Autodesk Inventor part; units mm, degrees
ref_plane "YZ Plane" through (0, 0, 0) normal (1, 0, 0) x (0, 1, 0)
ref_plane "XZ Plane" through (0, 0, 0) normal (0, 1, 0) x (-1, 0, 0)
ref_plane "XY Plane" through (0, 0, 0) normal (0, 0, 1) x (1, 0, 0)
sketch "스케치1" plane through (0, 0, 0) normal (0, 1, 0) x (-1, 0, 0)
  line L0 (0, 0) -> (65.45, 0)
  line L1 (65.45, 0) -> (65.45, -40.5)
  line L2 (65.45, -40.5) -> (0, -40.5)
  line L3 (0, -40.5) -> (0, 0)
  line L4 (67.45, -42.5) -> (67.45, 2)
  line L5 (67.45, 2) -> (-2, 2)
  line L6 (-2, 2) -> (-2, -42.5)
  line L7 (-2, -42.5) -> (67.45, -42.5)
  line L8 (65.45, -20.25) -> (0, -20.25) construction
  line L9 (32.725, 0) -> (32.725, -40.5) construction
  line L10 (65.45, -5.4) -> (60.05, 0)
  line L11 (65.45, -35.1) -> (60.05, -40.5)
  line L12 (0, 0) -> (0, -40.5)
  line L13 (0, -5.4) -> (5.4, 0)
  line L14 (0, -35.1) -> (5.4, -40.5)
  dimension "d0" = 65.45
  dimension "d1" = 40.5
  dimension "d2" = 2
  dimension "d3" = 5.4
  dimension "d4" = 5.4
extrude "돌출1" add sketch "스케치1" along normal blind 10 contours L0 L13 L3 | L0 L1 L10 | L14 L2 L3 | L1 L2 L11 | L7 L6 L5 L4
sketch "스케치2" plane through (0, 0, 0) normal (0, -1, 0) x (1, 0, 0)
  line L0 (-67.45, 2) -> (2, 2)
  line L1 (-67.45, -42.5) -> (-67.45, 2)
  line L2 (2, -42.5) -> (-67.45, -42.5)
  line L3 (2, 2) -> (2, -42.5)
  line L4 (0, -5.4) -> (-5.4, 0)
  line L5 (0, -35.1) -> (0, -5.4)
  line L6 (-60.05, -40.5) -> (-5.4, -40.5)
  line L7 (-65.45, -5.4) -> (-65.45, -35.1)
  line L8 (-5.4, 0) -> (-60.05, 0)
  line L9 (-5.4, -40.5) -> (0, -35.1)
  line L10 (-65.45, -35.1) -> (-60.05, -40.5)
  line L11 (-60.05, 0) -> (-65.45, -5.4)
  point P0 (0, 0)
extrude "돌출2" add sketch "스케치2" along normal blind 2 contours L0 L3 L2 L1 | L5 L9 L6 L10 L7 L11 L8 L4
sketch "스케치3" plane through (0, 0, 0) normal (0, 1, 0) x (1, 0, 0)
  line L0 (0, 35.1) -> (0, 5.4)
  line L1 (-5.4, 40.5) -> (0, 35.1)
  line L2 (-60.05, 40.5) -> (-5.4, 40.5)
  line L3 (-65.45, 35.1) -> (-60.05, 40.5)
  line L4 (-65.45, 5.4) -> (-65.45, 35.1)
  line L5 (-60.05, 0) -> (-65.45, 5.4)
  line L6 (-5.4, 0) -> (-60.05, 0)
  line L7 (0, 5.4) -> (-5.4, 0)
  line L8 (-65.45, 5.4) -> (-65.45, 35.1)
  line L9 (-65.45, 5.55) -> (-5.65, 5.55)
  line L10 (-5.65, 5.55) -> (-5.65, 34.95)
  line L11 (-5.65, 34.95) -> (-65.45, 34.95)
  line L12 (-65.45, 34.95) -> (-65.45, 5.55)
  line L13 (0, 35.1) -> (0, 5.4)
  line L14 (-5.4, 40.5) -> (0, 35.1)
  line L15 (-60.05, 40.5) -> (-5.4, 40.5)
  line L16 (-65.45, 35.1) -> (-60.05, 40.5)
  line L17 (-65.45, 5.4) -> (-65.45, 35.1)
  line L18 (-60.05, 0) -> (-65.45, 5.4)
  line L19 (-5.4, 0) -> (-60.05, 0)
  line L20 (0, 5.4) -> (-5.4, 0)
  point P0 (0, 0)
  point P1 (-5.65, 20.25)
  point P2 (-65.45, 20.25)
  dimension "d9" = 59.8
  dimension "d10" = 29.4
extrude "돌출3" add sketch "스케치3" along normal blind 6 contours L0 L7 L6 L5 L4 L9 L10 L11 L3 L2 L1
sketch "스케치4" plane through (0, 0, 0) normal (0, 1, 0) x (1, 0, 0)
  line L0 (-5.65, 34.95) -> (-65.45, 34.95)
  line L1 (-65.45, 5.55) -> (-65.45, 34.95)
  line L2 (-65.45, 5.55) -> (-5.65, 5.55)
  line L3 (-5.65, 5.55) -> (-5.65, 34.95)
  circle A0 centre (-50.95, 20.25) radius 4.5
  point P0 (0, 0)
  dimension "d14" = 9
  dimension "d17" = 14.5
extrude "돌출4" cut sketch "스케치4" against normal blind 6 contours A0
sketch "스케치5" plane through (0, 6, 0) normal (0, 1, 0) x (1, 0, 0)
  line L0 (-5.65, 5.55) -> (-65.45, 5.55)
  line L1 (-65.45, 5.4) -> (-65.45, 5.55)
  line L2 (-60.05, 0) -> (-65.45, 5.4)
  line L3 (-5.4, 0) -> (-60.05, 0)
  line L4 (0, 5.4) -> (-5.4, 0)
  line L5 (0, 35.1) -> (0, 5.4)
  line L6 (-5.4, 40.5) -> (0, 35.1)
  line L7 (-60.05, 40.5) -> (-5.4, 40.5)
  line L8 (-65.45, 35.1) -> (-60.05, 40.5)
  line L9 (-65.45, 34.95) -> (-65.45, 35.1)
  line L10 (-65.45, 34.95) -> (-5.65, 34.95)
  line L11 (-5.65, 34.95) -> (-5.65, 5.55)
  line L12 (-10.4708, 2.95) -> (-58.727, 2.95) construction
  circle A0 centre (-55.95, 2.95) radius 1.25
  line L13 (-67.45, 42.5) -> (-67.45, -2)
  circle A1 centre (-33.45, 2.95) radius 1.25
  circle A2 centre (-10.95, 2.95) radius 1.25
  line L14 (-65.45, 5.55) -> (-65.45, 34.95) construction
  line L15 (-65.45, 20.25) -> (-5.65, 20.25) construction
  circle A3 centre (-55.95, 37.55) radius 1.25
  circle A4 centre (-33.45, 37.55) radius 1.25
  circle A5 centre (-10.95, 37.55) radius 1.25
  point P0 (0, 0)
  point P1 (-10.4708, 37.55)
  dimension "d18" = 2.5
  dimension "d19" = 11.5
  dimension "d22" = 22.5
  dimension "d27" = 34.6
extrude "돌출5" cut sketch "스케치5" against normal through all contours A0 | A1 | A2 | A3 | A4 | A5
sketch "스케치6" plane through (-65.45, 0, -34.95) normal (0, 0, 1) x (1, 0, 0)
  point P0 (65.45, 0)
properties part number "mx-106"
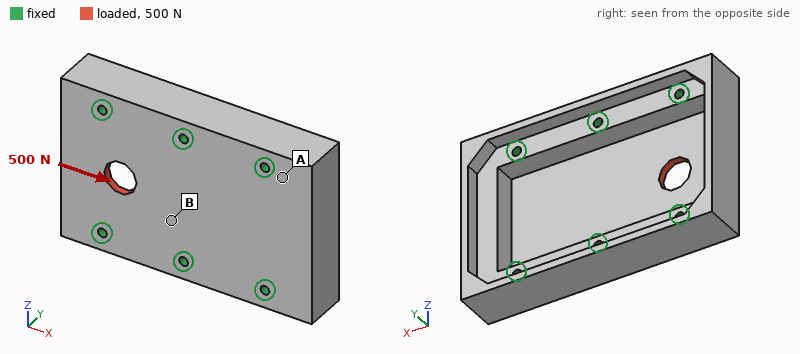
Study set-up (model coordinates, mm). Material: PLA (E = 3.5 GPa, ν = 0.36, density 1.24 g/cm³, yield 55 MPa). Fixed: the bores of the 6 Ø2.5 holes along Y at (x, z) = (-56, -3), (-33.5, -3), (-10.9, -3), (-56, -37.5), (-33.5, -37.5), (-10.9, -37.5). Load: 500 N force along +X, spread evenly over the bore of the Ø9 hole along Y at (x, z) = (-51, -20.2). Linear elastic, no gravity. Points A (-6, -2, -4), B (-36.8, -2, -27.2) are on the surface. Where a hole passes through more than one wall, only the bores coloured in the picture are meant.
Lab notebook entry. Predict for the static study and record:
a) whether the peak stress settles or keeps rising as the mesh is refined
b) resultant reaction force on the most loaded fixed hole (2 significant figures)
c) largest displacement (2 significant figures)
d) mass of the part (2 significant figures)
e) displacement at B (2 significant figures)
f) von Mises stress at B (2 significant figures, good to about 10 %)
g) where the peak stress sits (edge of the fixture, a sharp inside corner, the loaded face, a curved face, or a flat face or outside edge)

keeps rising
130 N
56 µm
20 g
16 µm
4.3 MPa
a sharp inside corner
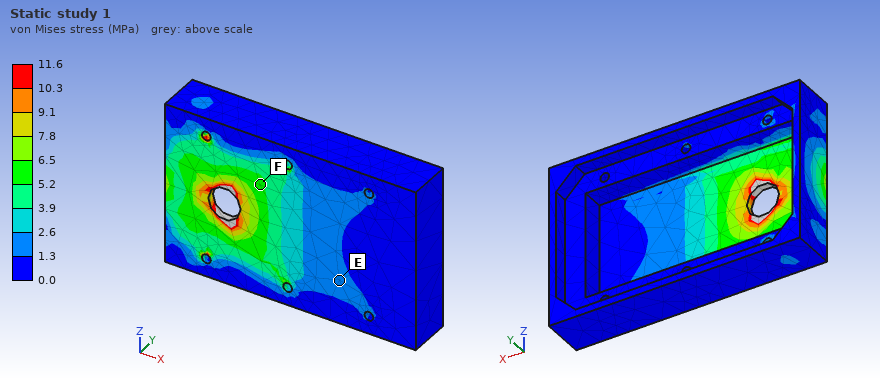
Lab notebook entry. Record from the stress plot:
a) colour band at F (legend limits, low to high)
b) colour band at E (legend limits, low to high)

5.2 to 6.5 MPa
1.3 to 2.6 MPa
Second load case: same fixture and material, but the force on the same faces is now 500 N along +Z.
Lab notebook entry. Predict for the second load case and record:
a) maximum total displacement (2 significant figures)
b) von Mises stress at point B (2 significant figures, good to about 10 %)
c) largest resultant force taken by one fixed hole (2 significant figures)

35 µm
2.0 MPa
180 N
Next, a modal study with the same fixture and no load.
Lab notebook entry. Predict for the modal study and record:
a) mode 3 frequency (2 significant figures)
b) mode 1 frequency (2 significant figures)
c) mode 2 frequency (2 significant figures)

4900 Hz
3900 Hz
4700 Hz
